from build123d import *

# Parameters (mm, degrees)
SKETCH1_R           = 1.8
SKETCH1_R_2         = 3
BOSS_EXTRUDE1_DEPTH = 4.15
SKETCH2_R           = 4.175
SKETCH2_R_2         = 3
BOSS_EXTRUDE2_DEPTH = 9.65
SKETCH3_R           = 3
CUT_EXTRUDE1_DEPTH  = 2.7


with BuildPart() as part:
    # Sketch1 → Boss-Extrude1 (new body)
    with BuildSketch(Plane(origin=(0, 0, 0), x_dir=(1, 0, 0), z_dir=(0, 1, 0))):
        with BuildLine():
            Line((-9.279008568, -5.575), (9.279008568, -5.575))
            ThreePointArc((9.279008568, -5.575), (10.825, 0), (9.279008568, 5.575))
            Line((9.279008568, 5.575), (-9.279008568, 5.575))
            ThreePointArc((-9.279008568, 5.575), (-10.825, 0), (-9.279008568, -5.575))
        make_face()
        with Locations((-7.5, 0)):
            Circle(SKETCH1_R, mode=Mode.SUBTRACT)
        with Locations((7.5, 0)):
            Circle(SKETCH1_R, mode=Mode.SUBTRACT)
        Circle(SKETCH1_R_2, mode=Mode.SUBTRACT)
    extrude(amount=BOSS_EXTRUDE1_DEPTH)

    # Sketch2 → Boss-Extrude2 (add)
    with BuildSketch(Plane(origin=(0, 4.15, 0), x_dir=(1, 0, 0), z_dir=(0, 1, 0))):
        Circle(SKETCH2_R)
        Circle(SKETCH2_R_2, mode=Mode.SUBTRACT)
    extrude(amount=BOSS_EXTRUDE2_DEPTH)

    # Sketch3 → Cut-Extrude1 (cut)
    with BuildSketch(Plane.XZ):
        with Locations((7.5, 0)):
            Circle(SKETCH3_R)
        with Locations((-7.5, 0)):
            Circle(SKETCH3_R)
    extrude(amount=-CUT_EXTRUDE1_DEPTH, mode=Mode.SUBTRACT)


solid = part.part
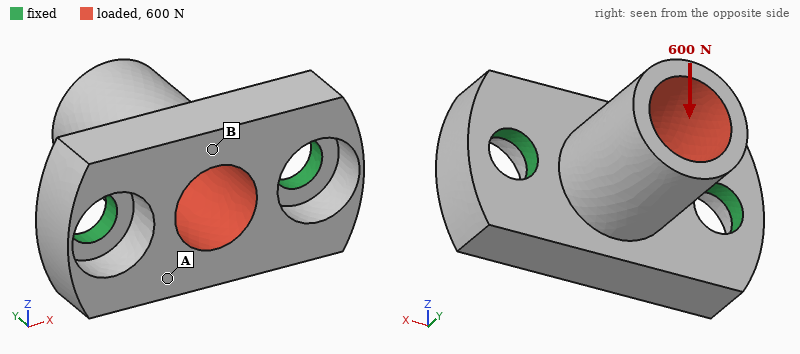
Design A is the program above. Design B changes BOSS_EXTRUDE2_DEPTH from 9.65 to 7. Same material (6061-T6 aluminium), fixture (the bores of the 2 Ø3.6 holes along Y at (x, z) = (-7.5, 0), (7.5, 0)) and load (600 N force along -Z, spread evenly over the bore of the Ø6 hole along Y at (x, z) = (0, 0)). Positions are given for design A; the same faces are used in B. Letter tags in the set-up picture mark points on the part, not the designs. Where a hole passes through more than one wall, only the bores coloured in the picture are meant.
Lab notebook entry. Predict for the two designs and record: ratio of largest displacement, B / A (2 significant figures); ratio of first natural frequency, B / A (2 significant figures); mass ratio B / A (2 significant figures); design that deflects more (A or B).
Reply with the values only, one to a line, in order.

0.52
1.3
0.92
A
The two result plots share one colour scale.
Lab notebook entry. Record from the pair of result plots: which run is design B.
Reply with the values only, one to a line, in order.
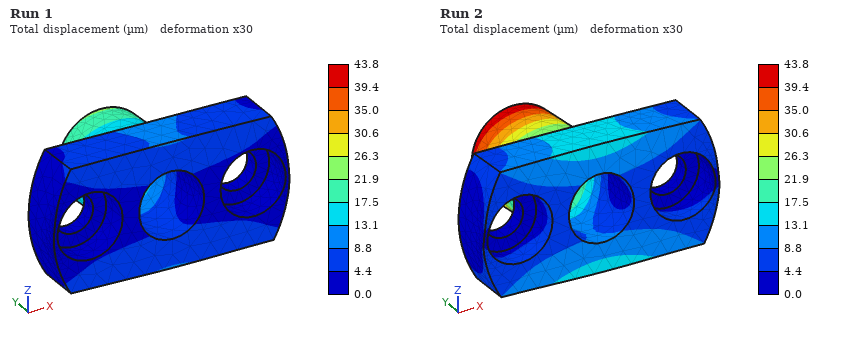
Run 1
